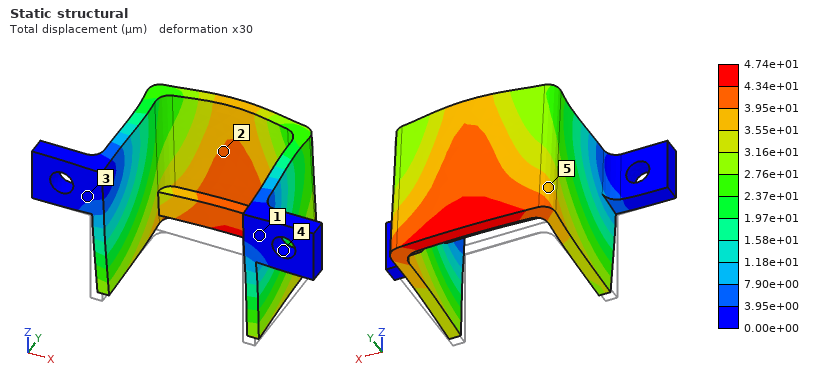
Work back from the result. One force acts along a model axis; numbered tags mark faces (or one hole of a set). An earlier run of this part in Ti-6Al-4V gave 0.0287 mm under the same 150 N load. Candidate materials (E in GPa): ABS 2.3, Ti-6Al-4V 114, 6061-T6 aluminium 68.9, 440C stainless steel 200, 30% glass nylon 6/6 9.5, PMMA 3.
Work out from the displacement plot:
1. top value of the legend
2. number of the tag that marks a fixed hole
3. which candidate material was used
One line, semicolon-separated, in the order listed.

4.74e+01 µm; 4; 6061-T6 aluminium
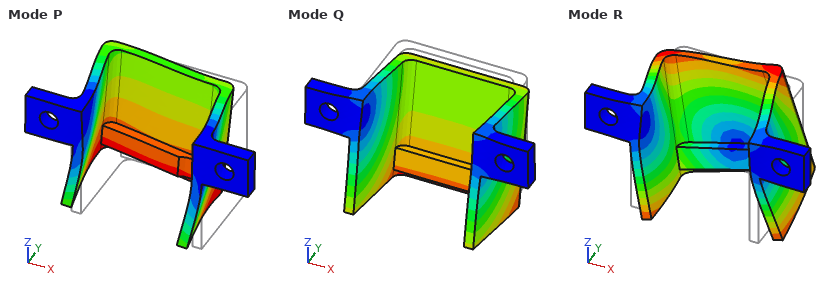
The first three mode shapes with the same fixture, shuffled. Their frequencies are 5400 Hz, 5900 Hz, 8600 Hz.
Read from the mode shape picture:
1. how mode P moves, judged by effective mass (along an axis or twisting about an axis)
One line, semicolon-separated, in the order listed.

along X
